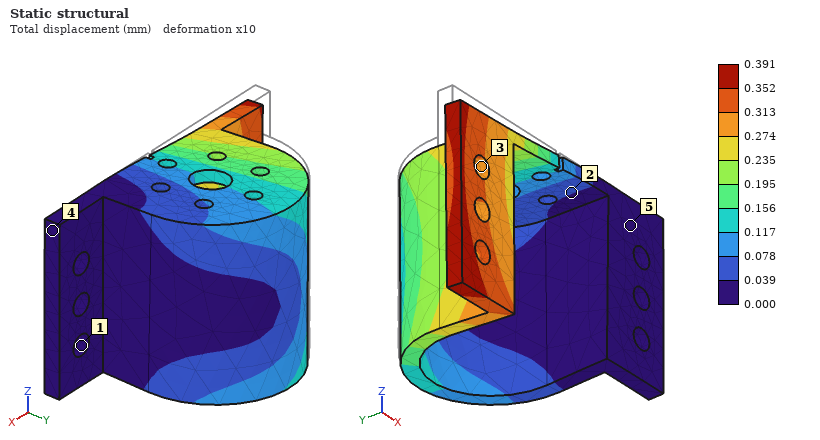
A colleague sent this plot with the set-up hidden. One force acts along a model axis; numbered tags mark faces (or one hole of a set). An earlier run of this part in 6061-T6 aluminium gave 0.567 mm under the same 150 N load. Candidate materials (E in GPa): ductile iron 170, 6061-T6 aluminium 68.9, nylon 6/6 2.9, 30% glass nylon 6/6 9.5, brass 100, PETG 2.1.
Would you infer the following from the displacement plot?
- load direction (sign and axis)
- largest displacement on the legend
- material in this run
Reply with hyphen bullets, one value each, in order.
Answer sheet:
- -Z
- 0.391 mm
- brass
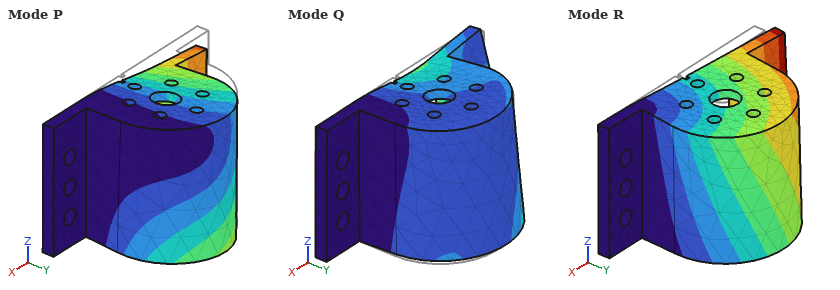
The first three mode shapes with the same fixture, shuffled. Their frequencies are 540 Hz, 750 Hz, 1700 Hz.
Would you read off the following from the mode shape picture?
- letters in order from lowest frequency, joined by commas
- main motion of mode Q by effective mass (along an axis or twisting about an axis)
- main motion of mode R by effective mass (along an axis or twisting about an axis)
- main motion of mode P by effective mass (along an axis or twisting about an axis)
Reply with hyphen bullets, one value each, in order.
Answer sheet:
- R, P, Q
- along X
- along Y
- along Z
